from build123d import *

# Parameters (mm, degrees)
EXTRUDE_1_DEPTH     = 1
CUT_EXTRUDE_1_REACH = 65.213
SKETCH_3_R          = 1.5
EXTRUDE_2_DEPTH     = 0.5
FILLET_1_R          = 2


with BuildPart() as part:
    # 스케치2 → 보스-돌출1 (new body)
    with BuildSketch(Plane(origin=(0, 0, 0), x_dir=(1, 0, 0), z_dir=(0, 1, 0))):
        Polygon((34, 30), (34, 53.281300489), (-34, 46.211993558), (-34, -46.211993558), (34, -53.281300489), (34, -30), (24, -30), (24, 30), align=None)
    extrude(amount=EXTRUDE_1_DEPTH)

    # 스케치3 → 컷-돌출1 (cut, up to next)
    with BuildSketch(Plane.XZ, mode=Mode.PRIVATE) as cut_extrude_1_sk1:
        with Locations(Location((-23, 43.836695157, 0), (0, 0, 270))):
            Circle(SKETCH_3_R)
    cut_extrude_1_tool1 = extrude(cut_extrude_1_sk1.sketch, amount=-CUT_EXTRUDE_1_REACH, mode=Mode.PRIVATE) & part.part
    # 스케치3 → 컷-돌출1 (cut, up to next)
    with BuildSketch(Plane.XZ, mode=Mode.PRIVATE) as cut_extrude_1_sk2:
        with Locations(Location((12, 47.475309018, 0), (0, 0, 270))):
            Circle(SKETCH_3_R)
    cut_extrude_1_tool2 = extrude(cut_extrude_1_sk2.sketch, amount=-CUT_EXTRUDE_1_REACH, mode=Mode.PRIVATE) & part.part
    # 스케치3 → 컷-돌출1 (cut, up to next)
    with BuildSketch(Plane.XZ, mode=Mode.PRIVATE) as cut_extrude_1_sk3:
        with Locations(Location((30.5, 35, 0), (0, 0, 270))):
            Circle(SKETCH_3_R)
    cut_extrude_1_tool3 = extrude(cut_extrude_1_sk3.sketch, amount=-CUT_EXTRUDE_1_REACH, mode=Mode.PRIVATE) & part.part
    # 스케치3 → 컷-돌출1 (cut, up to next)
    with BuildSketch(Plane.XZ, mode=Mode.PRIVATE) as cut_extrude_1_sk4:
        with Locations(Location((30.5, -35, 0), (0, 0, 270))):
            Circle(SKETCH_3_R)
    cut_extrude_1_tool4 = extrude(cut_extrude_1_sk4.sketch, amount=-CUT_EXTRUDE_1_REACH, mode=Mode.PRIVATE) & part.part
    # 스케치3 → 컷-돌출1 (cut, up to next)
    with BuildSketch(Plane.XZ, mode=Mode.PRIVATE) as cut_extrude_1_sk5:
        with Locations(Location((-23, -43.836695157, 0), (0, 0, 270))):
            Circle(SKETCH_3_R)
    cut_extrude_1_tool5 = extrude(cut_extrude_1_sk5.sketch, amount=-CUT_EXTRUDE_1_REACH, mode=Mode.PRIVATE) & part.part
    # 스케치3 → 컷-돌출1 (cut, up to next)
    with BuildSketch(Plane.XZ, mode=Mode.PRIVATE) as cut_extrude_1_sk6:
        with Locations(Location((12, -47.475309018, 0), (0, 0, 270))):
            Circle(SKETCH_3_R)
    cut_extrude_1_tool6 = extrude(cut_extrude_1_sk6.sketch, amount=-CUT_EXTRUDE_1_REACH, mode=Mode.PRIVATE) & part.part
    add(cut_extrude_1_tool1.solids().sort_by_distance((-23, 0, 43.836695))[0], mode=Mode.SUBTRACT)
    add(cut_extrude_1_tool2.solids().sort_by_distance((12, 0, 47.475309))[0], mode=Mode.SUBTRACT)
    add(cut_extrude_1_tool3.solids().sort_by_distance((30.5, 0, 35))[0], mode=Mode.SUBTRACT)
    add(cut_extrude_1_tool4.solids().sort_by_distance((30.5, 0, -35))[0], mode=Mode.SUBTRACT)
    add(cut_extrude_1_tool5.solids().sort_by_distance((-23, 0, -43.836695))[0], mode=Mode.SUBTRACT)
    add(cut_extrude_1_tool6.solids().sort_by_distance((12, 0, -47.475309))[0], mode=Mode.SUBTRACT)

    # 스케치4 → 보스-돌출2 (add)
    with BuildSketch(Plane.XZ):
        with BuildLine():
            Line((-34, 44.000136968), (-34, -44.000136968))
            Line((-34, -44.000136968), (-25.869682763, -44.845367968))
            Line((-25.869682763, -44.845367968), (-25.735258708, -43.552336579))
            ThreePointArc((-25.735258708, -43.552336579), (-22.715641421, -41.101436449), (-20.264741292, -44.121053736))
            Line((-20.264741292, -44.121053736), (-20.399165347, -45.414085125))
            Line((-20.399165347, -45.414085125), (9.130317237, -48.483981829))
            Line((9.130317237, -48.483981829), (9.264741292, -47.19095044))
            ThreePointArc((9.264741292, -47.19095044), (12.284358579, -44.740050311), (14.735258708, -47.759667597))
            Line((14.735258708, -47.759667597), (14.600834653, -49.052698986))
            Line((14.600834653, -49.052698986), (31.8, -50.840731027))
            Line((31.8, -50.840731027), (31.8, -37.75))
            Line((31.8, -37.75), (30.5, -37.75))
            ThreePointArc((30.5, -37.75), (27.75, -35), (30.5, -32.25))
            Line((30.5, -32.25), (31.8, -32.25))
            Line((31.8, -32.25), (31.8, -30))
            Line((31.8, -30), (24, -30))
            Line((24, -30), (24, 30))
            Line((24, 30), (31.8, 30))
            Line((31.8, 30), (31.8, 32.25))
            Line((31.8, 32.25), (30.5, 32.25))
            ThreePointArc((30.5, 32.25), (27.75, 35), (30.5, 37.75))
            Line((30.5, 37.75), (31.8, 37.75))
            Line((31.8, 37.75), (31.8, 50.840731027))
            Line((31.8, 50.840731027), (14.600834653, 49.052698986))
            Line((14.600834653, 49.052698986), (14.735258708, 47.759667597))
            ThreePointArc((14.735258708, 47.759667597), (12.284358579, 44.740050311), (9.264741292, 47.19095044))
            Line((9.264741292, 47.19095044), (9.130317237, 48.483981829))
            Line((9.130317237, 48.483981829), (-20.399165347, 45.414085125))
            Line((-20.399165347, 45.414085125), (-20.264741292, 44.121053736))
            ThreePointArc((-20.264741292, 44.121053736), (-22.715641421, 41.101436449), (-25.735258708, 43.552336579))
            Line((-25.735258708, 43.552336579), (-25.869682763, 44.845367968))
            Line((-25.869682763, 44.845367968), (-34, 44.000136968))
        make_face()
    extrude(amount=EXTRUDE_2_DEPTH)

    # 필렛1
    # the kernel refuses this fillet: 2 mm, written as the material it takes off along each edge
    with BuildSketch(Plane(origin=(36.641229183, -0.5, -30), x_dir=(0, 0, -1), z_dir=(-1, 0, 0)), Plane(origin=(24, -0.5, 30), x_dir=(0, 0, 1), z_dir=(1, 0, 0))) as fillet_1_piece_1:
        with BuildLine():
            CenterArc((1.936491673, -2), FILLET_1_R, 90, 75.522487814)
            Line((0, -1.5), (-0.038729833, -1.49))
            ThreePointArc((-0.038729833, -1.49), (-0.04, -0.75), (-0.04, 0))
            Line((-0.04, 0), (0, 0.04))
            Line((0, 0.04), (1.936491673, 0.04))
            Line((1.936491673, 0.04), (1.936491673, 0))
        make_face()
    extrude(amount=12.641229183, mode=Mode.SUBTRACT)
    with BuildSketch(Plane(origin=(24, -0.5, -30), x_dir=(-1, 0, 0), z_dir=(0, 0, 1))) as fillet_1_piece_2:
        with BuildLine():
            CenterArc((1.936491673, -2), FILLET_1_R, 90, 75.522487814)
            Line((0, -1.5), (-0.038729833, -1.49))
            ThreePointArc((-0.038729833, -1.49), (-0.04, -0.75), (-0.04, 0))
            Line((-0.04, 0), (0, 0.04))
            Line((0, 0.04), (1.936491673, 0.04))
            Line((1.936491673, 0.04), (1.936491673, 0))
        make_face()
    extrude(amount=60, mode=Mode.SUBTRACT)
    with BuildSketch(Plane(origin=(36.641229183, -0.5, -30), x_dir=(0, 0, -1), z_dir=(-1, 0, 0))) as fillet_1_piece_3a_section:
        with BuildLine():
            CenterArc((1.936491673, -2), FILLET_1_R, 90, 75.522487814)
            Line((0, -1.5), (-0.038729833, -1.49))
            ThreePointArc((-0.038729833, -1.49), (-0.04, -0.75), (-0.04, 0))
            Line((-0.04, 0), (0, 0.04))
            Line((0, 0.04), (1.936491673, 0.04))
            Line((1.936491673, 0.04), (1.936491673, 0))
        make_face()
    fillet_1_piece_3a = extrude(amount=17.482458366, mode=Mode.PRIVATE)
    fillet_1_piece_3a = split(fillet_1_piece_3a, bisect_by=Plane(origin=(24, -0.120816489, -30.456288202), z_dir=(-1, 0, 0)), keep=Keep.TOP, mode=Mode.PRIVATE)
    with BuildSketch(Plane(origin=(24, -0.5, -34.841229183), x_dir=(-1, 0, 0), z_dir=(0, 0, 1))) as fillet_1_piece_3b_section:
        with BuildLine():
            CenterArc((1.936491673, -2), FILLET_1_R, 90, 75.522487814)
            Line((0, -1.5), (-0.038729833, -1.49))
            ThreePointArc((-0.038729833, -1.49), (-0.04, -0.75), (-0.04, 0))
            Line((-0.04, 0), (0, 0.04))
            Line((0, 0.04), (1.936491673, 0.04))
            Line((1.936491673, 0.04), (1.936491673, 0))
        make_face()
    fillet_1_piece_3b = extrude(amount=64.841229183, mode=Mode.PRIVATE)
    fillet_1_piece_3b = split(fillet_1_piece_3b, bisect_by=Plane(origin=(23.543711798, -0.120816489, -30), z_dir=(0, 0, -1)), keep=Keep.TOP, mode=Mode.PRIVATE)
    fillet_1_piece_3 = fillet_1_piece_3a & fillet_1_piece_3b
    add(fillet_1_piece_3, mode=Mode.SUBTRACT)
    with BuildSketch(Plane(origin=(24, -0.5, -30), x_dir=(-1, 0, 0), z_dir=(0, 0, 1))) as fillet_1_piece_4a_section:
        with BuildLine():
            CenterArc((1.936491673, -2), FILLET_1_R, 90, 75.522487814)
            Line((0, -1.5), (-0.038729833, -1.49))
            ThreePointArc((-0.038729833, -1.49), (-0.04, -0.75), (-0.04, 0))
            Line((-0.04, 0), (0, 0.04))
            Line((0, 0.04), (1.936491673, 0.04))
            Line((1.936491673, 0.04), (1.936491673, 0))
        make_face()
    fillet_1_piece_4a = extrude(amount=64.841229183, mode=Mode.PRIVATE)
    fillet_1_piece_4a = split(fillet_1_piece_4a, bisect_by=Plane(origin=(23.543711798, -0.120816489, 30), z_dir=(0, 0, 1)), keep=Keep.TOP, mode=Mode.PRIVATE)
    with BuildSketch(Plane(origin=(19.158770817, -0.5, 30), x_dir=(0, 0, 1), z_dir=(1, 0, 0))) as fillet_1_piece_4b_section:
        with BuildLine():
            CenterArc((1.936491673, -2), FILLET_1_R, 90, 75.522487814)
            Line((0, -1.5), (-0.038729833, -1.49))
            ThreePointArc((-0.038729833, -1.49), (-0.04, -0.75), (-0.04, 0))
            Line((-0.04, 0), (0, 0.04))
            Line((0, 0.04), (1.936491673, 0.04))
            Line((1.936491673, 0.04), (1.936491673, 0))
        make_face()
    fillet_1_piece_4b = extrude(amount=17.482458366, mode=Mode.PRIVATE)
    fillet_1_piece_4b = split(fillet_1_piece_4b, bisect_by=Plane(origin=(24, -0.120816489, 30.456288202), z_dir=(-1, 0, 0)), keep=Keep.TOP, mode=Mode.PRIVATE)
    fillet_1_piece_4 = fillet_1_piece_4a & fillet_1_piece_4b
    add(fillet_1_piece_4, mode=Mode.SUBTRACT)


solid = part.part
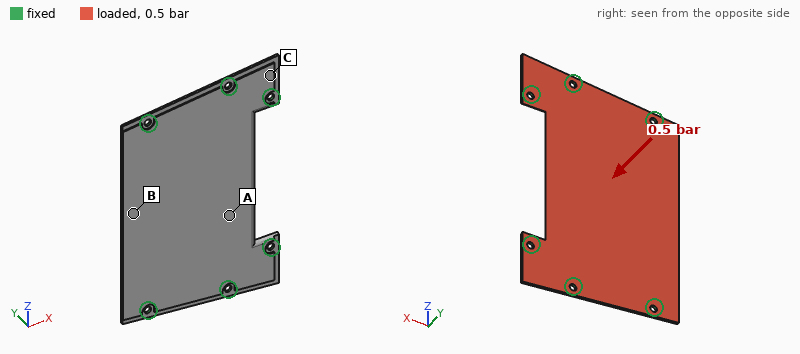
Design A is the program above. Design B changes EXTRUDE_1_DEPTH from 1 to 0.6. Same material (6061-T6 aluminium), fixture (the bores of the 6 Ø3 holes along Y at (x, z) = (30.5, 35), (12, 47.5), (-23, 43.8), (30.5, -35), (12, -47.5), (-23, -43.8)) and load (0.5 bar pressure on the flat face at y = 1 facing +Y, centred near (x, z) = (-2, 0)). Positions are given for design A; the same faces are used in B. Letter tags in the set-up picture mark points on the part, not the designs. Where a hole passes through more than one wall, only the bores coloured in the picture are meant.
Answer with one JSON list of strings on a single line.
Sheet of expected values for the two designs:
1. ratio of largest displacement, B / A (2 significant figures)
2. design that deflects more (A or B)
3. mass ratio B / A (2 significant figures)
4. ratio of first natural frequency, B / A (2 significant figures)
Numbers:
["2.7", "B", "0.72", "0.71"]
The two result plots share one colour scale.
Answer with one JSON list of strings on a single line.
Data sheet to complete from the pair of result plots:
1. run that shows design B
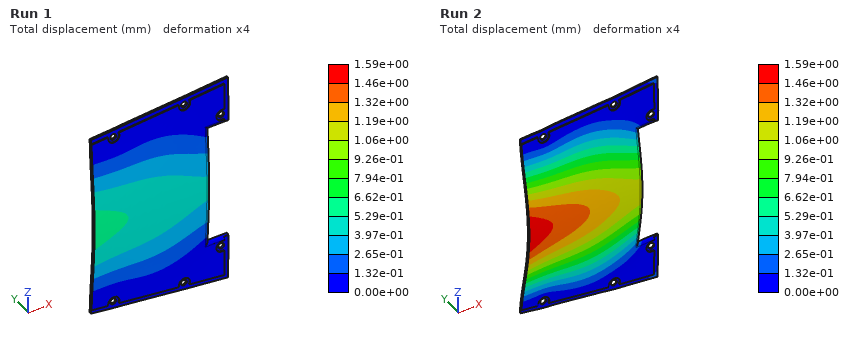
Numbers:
["Run 2"]
